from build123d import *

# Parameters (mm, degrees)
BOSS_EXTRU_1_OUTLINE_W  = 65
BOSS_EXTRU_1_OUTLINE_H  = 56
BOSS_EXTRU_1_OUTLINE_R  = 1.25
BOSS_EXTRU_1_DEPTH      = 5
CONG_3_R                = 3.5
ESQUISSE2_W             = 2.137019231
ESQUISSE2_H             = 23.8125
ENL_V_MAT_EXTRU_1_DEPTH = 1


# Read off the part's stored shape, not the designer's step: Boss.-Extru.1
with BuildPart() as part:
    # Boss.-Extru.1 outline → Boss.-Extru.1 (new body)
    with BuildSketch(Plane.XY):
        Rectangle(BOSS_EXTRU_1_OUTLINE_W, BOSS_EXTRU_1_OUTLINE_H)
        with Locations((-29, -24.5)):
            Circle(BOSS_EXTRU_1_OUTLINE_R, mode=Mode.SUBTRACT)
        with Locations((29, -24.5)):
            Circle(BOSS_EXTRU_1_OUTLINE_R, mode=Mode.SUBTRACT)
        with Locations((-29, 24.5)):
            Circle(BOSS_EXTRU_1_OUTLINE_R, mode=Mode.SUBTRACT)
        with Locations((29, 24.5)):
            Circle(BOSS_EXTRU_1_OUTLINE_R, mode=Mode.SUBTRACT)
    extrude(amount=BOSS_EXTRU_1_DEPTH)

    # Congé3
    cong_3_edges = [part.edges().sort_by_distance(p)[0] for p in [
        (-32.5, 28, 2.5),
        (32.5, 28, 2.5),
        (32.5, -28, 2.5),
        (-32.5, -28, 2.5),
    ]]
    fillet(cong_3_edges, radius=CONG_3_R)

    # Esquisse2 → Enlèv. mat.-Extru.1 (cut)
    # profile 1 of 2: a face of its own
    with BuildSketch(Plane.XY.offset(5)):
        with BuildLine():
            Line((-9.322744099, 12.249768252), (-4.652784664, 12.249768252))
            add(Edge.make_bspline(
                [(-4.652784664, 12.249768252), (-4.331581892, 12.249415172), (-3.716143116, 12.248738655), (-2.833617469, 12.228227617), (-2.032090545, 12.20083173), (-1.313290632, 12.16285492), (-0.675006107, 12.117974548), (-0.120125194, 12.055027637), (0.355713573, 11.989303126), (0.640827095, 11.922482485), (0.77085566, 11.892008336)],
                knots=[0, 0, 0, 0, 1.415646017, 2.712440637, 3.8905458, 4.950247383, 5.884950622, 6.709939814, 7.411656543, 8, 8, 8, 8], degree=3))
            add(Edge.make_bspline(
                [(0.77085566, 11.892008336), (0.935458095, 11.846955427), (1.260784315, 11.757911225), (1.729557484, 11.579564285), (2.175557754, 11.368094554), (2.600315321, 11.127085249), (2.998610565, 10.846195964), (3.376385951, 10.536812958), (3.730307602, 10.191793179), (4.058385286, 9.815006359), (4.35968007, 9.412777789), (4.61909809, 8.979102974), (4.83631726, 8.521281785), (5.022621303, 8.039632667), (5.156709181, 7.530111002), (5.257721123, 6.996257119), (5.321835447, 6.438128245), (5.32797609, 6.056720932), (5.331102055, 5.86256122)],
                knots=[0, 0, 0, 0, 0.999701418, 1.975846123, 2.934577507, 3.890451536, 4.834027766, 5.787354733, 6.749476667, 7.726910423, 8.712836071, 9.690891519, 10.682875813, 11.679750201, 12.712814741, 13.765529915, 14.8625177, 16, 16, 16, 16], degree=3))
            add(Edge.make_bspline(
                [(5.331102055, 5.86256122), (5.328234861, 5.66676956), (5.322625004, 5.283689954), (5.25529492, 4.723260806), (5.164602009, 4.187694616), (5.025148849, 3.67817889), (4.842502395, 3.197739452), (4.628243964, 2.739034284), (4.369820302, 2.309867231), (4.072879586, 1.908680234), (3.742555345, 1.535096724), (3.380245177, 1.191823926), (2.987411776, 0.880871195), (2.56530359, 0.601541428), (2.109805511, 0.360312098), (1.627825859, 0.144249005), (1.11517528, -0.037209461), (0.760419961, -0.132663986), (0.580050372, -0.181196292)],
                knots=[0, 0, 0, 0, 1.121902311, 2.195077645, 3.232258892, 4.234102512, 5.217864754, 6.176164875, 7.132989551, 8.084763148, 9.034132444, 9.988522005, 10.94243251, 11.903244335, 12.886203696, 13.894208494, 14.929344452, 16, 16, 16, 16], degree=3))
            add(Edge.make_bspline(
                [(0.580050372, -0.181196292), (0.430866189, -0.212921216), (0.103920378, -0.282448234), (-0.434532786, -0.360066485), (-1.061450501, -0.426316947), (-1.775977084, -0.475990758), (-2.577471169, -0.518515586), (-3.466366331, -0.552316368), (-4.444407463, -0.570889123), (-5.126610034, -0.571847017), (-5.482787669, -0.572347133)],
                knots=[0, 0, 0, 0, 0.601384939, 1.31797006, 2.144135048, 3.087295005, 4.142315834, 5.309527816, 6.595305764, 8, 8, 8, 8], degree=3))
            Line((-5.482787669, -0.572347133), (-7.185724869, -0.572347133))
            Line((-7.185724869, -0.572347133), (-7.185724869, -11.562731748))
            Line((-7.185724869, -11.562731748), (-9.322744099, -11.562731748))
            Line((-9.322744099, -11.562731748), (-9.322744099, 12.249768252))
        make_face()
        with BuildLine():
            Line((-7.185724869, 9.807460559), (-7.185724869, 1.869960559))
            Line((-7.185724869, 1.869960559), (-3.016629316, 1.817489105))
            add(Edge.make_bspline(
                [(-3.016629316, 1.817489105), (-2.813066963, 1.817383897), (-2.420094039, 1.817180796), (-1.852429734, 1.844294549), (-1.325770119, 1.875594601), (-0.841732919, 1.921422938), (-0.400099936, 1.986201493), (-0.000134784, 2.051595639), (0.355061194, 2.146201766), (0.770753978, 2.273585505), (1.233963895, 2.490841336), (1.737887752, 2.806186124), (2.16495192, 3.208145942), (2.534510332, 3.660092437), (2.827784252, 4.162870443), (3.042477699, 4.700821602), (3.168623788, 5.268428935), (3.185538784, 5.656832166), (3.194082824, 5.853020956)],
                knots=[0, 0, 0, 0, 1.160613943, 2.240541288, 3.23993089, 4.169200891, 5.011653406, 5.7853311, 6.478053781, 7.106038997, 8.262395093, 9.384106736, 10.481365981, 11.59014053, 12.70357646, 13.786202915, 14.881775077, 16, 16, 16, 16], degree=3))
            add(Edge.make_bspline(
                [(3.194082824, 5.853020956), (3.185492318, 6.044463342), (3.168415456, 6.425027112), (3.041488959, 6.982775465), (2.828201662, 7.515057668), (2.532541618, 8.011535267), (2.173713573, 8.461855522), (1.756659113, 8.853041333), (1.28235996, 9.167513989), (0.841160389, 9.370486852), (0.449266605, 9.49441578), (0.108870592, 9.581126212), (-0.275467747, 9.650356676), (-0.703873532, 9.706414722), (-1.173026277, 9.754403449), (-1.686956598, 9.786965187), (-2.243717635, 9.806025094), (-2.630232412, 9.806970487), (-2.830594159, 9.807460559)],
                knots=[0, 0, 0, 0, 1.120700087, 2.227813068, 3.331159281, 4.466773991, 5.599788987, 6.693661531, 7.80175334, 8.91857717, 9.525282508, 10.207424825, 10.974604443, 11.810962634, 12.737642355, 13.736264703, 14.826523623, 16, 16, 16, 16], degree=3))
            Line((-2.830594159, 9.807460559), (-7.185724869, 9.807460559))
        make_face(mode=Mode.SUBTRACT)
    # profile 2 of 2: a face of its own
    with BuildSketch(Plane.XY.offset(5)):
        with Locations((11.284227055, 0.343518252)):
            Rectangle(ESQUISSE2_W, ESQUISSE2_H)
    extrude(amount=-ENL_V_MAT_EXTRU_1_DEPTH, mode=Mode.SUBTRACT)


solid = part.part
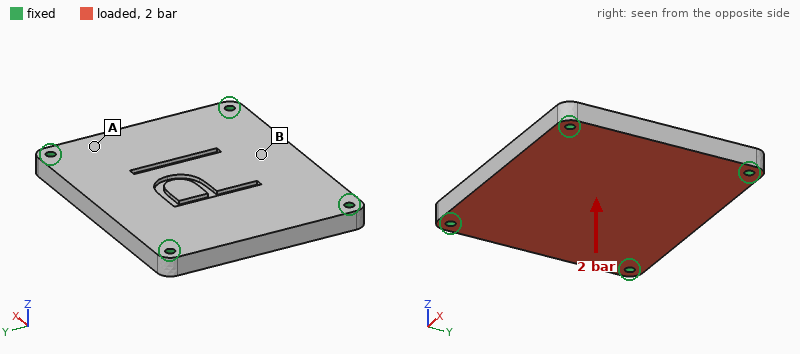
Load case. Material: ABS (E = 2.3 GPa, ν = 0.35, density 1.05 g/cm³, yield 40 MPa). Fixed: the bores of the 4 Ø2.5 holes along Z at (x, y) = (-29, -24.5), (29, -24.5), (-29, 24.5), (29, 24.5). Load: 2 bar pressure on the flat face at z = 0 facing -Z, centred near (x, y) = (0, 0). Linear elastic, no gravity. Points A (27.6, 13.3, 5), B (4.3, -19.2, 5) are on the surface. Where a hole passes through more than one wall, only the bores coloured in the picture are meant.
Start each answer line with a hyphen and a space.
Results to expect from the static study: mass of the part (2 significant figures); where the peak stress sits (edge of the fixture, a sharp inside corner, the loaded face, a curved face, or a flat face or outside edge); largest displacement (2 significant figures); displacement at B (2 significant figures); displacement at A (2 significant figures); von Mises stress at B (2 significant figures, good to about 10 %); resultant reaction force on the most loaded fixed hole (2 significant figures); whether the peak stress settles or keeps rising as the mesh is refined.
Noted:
- 19 g
- edge of the fixture
- 0.66 mm
- 0.50 mm
- 0.18 mm
- 9.2 MPa
- 180 N
- keeps rising
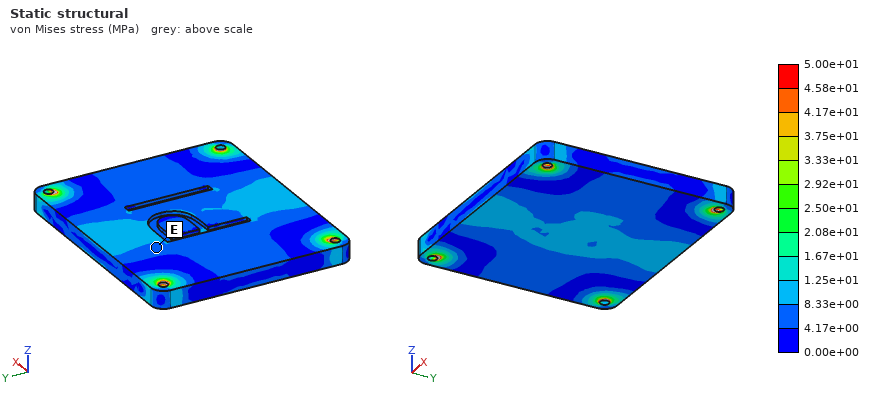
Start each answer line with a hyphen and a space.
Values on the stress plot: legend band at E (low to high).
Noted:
- 4.17e+00 to 8.33e+00 MPa
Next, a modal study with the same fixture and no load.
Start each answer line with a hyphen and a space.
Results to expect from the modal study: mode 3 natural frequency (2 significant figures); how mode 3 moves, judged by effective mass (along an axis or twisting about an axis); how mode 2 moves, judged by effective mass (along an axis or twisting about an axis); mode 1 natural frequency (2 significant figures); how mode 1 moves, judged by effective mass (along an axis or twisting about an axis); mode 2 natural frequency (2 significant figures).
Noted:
- 2900 Hz
- twisting about Y
- twisting about X
- 1500 Hz
- along Z
- 2400 Hz
